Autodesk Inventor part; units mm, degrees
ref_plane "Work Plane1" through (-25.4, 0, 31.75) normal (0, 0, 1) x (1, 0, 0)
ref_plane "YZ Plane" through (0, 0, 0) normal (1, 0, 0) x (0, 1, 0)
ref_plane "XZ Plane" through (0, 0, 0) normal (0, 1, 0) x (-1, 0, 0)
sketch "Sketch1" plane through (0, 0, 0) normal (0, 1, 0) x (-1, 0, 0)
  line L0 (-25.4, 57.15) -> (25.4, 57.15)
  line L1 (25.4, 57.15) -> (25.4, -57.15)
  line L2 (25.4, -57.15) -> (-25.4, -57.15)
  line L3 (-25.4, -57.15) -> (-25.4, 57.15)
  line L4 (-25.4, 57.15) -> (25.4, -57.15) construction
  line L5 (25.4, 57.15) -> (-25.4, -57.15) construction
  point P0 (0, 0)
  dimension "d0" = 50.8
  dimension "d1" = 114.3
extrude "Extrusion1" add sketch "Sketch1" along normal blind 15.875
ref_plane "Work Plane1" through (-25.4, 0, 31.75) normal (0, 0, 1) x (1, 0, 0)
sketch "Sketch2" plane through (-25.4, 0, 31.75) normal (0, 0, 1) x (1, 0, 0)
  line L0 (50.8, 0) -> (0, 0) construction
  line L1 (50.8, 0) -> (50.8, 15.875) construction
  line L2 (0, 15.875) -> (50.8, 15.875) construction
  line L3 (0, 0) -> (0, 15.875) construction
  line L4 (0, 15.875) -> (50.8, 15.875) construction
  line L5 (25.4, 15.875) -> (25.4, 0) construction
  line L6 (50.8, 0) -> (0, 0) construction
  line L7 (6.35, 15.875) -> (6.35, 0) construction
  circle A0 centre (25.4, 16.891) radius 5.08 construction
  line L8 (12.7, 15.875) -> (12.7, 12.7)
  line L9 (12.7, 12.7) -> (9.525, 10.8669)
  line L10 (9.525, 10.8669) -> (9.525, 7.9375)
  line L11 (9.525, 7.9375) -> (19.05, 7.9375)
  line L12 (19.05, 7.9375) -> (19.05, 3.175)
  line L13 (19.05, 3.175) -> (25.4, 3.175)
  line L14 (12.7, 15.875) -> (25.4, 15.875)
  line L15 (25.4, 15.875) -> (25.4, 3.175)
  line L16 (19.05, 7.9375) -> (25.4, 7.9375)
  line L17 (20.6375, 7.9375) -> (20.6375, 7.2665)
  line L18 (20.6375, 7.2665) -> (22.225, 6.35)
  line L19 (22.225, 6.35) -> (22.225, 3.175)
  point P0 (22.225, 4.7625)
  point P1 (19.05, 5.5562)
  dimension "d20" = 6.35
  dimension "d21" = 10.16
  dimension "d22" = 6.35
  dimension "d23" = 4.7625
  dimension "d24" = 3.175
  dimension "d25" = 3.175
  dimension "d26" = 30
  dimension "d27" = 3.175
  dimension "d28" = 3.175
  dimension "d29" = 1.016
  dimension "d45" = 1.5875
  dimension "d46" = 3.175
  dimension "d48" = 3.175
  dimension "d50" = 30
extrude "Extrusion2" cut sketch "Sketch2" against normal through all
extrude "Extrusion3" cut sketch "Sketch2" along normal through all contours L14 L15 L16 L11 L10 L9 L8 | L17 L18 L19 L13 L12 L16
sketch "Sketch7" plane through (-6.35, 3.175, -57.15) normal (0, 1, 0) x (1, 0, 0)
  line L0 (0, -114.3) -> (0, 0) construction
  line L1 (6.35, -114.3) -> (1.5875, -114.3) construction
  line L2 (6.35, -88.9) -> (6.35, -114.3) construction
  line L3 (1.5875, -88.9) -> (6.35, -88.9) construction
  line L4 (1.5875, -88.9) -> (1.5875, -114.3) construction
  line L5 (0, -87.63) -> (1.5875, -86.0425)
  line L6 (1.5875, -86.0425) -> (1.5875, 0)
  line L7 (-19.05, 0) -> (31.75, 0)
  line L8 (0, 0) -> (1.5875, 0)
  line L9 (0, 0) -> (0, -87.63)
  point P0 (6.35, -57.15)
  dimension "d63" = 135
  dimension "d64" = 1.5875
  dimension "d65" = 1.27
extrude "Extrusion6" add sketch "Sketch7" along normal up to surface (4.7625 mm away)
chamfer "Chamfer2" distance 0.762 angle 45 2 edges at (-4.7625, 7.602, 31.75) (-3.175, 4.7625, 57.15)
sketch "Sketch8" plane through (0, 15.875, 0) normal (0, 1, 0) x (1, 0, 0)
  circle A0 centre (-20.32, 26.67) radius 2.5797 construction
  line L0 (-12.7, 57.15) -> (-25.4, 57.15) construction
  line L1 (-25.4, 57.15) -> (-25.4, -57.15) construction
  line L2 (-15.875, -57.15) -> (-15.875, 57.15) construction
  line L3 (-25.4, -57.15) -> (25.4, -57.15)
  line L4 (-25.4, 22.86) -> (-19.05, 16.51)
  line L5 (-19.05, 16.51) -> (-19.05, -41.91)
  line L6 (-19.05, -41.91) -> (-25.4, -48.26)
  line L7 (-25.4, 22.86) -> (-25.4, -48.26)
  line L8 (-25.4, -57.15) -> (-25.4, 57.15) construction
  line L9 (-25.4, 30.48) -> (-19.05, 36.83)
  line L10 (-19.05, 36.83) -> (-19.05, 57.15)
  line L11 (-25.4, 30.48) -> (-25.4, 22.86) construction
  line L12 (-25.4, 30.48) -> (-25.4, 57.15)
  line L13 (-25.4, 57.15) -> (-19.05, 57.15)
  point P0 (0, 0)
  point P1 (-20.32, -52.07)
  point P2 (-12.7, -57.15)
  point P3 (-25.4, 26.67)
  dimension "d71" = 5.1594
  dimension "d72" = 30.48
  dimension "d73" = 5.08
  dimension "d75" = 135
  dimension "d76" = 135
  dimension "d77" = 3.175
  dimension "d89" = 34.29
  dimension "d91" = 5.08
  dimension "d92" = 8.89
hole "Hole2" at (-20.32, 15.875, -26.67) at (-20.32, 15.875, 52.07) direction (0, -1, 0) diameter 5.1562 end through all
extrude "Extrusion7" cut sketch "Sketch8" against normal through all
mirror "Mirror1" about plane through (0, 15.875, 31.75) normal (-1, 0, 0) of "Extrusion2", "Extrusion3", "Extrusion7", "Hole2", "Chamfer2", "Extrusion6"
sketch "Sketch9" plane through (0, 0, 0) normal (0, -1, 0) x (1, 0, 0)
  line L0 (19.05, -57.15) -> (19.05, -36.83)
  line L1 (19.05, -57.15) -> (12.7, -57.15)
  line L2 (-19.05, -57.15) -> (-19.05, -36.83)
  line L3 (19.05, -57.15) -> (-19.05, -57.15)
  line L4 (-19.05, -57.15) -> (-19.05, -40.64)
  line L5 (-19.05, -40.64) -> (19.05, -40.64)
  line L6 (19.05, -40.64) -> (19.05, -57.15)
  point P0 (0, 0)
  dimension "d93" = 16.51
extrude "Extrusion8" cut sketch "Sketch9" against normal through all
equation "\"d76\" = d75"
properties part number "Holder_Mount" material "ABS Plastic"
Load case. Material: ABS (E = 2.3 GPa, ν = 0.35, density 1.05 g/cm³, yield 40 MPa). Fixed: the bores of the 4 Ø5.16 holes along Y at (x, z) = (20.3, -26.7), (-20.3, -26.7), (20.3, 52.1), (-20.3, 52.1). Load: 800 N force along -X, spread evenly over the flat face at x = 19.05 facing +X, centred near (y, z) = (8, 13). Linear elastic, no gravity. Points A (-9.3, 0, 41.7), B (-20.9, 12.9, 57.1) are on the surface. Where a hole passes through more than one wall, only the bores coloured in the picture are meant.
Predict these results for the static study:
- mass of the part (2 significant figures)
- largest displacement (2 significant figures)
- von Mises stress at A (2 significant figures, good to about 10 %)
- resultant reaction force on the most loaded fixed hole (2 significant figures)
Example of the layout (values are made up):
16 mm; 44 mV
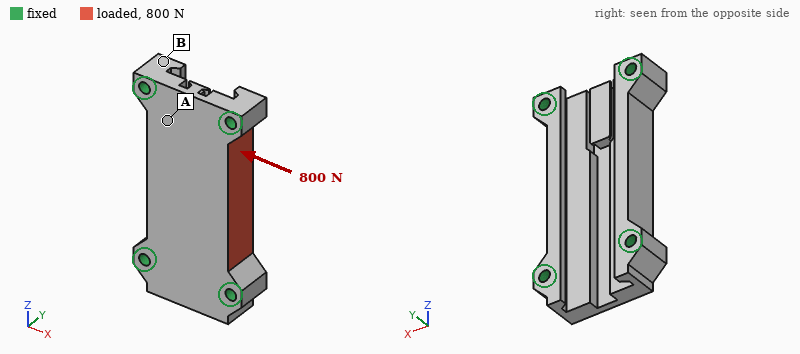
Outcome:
39 g; 0.35 mm; 3.4 MPa; 360 N
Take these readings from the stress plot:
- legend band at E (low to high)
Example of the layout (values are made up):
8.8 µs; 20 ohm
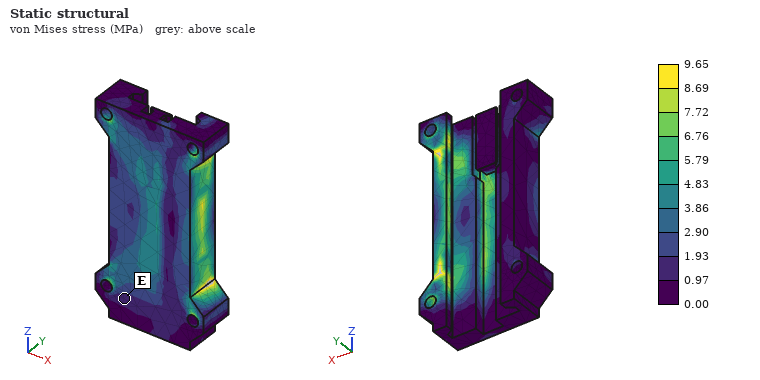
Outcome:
0.97 to 1.93 MPa
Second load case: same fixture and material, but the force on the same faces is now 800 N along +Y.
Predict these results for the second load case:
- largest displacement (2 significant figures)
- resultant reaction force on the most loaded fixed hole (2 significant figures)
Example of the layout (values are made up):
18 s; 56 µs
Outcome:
0.44 mm; 410 N
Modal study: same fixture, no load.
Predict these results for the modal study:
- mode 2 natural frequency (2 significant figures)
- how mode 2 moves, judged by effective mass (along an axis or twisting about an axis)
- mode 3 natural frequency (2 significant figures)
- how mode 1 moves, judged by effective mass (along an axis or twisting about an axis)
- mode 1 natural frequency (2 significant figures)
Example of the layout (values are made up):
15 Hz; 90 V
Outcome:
3200 Hz; along X; 3800 Hz; along Y; 2500 Hz
